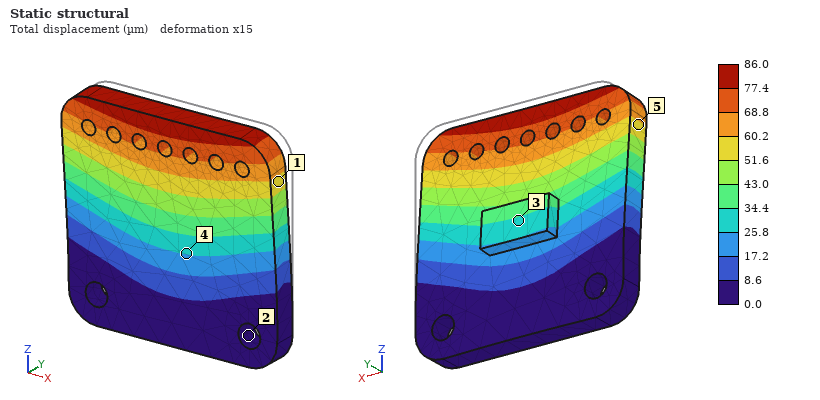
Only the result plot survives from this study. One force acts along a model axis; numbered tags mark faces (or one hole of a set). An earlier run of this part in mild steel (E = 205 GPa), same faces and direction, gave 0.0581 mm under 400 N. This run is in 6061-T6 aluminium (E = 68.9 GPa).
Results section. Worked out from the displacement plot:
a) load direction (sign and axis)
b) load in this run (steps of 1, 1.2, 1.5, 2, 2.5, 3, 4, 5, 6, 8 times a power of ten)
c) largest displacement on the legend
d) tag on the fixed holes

-Y
200 N
86.0 µm
2
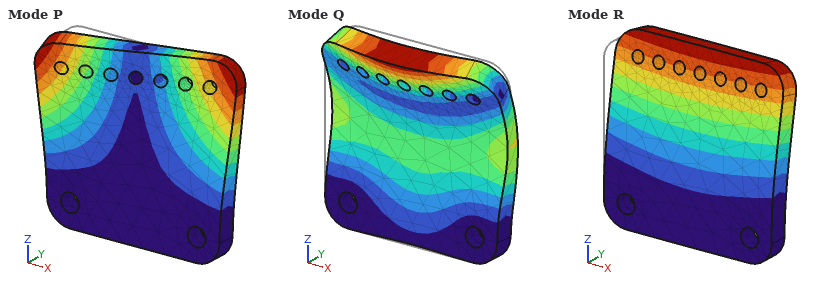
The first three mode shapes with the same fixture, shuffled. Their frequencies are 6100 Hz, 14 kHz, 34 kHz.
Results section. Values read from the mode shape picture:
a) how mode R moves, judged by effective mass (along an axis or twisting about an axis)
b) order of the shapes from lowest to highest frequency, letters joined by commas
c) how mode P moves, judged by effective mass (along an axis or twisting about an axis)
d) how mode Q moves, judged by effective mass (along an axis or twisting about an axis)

along Y
R, P, Q
twisting about Z
along Y
